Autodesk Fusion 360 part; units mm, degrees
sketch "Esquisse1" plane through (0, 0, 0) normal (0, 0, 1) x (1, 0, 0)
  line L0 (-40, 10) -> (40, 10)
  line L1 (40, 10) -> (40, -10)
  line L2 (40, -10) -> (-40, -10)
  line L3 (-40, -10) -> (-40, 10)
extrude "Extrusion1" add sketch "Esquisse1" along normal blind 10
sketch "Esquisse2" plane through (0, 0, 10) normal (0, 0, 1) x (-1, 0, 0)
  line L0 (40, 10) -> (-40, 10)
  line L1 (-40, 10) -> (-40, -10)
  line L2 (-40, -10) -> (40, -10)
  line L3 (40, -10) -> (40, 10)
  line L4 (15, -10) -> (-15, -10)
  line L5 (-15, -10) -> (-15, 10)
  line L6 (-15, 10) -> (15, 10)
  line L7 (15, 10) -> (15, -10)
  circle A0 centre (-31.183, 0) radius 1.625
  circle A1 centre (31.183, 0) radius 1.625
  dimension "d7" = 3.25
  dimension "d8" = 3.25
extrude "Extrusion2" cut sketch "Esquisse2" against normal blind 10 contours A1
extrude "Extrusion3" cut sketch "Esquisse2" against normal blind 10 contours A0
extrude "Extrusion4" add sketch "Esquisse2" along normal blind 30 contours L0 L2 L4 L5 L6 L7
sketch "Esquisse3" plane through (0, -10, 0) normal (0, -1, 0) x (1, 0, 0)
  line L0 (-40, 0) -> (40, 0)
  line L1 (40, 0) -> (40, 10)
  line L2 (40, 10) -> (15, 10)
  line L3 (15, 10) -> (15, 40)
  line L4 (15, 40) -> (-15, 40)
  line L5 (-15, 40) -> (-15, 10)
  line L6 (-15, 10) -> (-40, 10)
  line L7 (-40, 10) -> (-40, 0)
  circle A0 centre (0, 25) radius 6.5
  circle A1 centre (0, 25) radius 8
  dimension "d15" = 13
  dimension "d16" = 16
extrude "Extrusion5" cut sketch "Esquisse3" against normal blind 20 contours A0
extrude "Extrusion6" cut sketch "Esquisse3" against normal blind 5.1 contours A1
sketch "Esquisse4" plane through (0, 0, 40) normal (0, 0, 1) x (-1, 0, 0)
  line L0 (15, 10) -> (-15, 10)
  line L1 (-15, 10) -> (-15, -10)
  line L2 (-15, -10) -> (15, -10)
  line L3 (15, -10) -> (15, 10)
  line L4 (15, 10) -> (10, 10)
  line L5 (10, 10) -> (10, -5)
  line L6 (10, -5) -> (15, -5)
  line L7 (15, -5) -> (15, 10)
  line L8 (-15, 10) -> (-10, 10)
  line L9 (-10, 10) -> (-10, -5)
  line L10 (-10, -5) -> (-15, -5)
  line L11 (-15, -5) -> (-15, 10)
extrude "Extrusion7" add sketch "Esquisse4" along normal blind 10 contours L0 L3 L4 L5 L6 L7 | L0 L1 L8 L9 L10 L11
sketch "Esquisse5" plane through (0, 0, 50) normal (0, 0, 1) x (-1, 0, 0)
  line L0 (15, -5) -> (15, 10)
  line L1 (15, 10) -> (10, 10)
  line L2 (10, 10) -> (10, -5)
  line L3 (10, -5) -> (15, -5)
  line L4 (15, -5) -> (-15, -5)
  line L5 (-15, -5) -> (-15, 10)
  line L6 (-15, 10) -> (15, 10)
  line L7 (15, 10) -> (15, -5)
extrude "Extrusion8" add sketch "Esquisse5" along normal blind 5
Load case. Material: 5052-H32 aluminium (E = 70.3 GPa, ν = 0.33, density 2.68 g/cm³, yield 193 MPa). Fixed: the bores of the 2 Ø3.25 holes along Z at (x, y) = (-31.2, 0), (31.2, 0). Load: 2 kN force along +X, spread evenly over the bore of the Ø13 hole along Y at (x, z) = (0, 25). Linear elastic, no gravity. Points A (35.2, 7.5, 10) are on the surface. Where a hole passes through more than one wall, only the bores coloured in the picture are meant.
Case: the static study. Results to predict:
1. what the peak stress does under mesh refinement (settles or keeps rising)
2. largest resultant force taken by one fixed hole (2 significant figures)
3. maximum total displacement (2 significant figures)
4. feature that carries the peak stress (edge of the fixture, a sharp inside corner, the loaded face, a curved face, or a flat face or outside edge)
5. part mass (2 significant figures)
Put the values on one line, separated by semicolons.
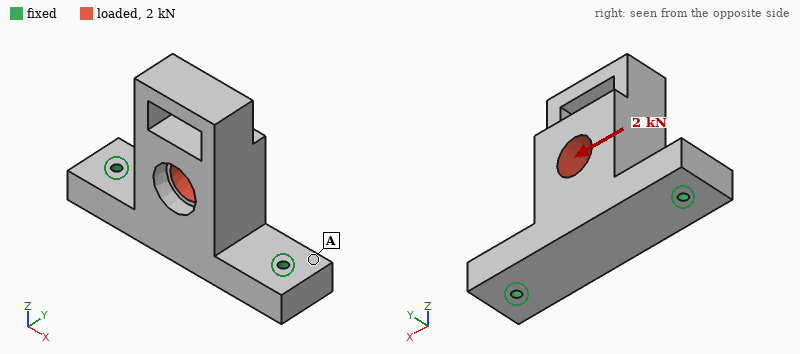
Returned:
keeps rising; 1.3 kN; 32 µm; edge of the fixture; 93 g
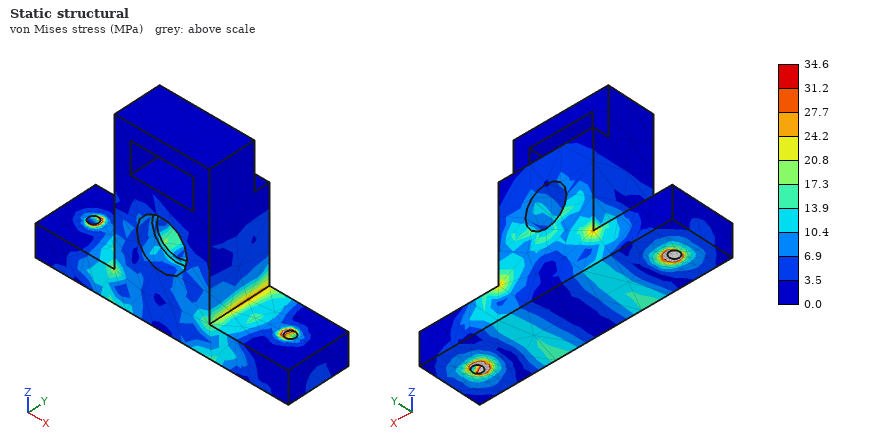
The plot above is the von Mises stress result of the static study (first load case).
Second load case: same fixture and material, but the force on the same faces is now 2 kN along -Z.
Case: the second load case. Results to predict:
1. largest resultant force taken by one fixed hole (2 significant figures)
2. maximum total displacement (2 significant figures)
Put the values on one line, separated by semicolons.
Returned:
1.1 kN; 29 µm
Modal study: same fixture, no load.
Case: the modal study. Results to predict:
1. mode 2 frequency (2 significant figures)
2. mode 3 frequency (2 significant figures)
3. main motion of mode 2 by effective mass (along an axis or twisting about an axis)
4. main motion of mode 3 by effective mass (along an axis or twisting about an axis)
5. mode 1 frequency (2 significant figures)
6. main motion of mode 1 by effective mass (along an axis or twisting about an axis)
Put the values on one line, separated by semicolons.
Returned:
5500 Hz; 7200 Hz; along X; along Z; 2400 Hz; along Y
